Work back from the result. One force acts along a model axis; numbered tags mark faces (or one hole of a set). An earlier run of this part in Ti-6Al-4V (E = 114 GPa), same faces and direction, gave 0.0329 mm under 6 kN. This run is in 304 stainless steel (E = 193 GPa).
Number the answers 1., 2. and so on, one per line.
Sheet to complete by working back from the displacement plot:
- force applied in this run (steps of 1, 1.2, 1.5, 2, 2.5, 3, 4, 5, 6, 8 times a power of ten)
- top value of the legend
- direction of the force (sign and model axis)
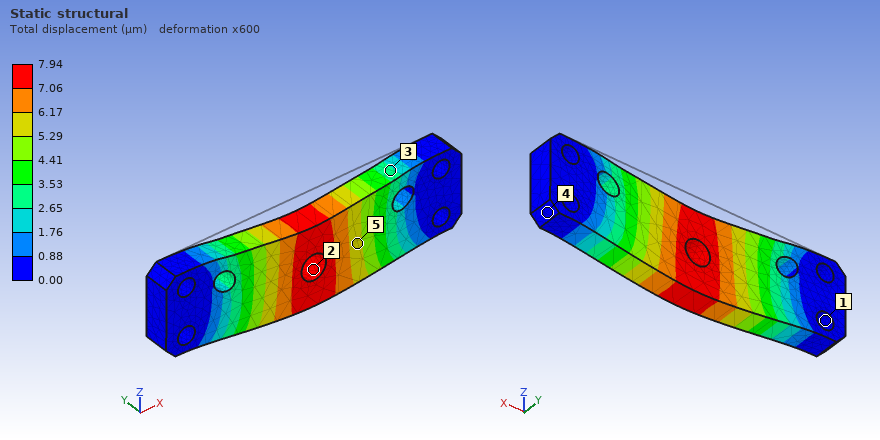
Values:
1. 2.5 kN
2. 7.94 µm
3. -Z
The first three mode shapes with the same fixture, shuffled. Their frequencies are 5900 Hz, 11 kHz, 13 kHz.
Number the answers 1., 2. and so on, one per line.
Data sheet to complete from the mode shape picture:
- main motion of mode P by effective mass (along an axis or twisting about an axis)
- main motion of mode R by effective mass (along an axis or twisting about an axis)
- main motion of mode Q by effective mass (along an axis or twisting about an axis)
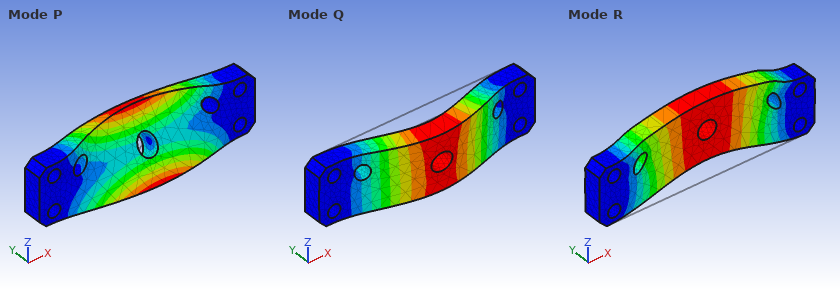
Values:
1. twisting about X
2. along Z
3. along Y
